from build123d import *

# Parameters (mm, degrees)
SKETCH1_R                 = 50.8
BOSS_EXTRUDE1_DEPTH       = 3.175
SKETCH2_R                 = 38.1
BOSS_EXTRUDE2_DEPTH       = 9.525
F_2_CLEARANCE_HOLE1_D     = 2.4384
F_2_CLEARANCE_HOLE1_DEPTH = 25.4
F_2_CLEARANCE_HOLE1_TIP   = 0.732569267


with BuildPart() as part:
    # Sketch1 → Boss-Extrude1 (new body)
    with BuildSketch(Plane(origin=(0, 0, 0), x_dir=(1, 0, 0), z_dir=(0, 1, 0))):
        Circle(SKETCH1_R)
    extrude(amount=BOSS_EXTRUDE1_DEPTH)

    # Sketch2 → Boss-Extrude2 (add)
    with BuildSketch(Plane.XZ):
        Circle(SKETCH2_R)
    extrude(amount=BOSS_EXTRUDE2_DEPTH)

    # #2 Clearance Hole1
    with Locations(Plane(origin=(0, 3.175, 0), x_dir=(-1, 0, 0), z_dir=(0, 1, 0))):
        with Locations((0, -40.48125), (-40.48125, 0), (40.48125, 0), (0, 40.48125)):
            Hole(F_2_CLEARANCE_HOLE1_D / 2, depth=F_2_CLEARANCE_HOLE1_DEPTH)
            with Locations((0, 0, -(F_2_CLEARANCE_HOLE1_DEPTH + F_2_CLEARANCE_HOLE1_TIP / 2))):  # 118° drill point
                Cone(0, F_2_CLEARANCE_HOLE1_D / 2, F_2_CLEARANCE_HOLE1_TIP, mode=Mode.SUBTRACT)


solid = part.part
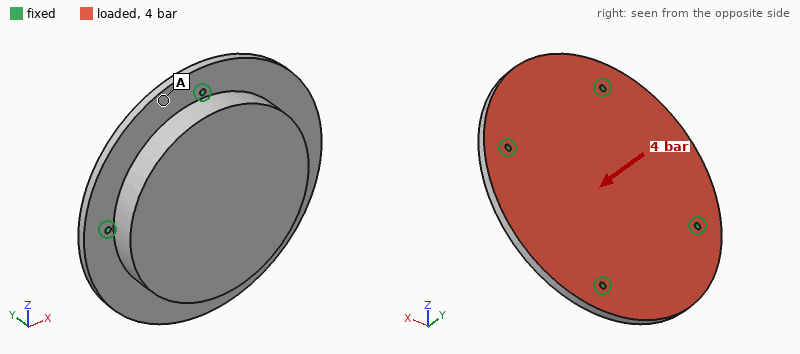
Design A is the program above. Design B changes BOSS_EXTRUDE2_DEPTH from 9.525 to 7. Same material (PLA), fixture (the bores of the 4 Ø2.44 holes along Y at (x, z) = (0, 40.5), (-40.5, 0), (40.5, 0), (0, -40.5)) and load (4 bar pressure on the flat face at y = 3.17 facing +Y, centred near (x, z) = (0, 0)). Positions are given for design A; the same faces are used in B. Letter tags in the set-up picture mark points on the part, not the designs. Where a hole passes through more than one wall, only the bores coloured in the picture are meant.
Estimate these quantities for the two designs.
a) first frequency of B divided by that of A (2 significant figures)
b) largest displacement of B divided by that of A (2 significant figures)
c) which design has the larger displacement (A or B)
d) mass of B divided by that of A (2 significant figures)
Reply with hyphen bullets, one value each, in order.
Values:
- 0.95
- 1.2
- B
- 0.83
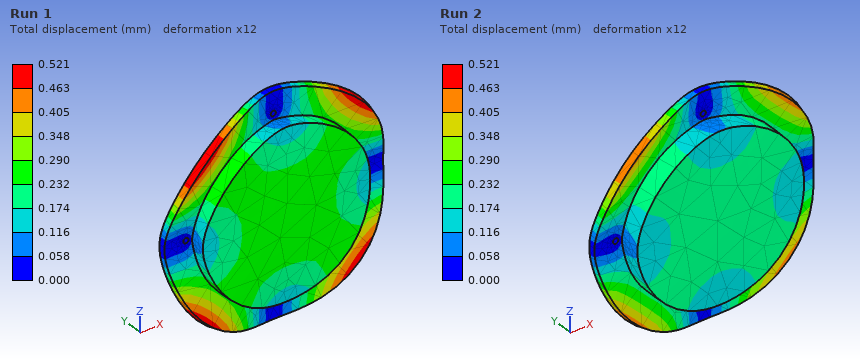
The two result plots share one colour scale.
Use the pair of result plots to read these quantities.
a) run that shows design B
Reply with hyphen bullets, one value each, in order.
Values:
- Run 1
